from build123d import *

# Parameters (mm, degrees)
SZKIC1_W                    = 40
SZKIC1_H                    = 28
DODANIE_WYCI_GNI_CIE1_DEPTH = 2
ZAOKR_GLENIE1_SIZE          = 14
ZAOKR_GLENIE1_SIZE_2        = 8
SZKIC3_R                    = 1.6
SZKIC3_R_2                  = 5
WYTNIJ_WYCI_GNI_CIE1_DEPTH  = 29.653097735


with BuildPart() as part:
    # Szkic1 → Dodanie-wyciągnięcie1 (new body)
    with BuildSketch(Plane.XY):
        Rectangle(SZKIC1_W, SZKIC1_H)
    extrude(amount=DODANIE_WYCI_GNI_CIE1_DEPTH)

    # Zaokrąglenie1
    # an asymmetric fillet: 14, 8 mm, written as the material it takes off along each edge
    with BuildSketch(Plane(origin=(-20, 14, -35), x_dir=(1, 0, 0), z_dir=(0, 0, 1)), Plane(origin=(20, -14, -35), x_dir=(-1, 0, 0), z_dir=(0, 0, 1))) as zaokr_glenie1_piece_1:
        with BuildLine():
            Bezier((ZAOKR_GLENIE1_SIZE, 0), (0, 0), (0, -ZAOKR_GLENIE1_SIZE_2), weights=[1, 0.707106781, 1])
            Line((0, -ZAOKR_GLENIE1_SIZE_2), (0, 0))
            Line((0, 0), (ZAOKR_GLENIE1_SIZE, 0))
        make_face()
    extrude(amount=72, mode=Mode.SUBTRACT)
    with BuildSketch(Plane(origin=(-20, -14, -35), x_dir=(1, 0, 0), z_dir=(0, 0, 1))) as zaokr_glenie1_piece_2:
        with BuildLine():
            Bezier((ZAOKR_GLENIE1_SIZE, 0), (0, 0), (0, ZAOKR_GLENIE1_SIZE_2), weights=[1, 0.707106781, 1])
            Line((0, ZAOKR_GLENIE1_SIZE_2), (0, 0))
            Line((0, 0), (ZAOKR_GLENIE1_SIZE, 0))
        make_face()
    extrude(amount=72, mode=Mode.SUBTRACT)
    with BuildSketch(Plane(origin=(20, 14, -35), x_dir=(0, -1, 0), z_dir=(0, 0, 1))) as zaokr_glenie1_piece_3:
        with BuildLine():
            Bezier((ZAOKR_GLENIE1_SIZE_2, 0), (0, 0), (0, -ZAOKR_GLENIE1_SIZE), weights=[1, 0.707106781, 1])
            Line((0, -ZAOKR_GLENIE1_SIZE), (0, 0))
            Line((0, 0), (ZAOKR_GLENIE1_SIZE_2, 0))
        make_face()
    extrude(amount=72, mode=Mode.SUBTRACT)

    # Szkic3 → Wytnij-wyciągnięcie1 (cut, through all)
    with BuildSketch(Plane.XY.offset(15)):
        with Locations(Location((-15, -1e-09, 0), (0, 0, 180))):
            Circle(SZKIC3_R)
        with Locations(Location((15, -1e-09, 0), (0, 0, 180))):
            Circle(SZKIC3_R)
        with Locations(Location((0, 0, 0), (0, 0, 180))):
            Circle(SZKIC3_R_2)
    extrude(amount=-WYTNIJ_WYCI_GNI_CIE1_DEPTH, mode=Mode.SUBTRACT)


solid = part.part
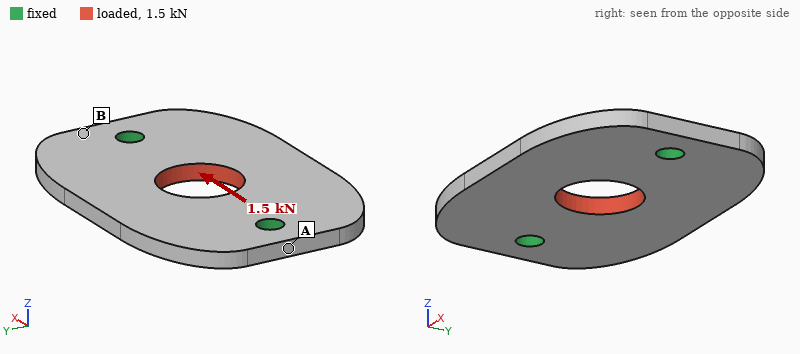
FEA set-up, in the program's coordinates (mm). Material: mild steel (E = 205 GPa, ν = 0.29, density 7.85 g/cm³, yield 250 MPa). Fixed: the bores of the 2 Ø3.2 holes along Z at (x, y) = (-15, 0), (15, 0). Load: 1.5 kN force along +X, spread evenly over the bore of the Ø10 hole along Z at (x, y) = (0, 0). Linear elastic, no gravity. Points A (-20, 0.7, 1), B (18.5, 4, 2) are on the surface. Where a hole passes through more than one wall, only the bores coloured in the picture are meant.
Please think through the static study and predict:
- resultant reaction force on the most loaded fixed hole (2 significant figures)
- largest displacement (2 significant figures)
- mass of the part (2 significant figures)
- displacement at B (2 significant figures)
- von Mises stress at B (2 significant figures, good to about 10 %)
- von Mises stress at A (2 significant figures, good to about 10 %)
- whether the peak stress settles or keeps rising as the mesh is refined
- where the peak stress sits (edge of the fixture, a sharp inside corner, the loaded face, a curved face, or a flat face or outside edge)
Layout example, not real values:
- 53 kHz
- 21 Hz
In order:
- 750 N
- 2.2 µm
- 15 g
- 0.58 µm
- 11 MPa
- 27 MPa
- keeps rising
- edge of the fixture
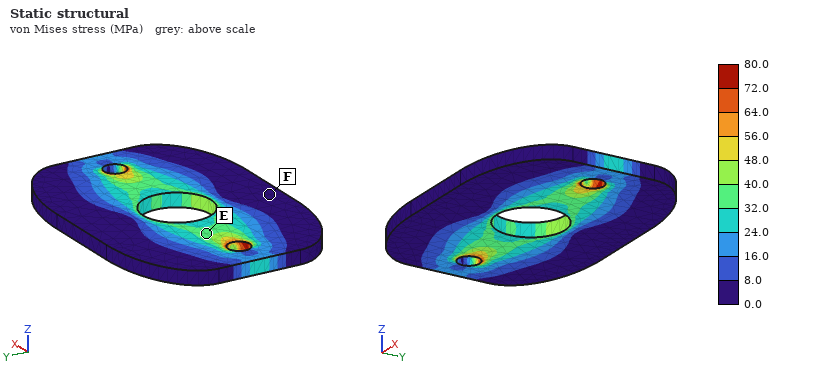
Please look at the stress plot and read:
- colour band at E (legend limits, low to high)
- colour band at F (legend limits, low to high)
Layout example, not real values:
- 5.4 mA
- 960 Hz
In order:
- 32.0 to 40.0 MPa
- 0.0 to 8.0 MPa
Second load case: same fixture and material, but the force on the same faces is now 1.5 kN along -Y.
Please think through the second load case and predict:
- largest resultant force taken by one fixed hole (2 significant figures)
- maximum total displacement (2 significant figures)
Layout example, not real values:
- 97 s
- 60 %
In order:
- 750 N
- 3.9 µm
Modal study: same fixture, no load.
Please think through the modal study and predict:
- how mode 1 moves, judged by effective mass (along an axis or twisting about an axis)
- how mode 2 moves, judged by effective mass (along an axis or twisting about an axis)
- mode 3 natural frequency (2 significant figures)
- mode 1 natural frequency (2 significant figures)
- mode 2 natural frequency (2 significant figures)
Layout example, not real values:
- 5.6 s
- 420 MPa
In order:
- twisting about X
- along Z
- 14 kHz
- 6500 Hz
- 7500 Hz
